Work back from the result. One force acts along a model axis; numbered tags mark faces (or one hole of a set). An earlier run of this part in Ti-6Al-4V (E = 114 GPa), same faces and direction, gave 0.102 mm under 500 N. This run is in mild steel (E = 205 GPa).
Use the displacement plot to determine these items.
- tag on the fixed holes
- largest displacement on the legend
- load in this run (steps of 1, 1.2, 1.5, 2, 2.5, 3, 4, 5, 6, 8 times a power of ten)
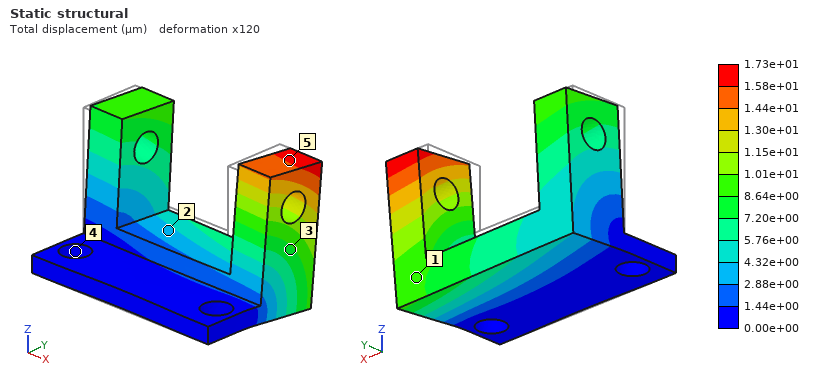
4
1.73e+01 µm
150 N
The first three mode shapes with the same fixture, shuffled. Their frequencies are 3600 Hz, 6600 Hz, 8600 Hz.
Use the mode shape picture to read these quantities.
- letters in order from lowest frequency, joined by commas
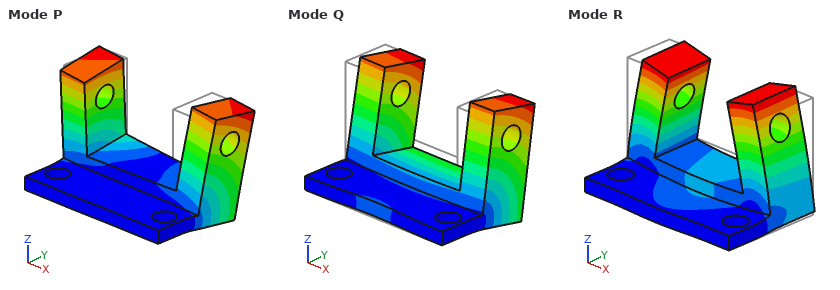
Q, P, R
